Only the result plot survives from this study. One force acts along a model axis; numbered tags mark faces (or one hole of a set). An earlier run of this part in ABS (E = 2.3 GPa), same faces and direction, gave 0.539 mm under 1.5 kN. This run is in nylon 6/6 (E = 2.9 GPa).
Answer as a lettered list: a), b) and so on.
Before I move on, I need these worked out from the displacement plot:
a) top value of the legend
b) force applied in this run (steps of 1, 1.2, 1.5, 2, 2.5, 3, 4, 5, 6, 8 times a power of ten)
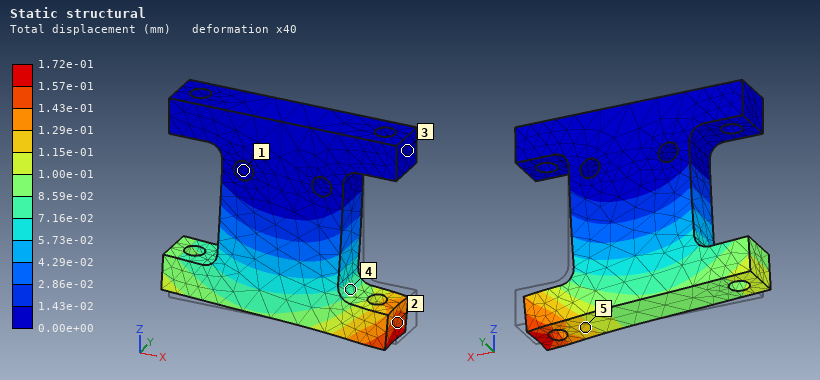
a) 1.72e-01 mm
b) 600 N
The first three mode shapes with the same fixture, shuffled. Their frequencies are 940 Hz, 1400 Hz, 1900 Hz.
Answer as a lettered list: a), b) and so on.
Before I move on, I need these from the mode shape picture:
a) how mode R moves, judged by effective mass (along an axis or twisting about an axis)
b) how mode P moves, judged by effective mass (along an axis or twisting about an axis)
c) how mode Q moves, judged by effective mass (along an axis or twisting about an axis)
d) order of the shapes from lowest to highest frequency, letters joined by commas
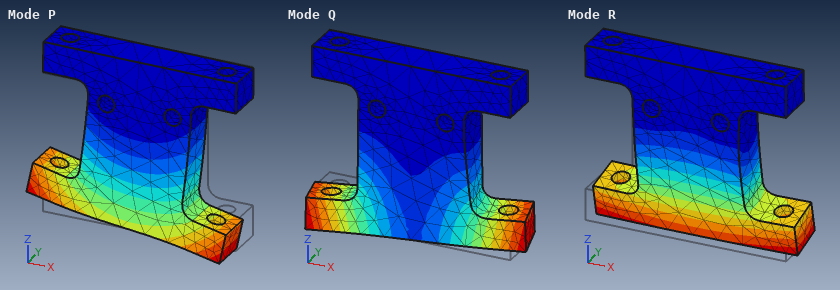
a) along Y
b) along X
c) twisting about Z
d) R, Q, P
